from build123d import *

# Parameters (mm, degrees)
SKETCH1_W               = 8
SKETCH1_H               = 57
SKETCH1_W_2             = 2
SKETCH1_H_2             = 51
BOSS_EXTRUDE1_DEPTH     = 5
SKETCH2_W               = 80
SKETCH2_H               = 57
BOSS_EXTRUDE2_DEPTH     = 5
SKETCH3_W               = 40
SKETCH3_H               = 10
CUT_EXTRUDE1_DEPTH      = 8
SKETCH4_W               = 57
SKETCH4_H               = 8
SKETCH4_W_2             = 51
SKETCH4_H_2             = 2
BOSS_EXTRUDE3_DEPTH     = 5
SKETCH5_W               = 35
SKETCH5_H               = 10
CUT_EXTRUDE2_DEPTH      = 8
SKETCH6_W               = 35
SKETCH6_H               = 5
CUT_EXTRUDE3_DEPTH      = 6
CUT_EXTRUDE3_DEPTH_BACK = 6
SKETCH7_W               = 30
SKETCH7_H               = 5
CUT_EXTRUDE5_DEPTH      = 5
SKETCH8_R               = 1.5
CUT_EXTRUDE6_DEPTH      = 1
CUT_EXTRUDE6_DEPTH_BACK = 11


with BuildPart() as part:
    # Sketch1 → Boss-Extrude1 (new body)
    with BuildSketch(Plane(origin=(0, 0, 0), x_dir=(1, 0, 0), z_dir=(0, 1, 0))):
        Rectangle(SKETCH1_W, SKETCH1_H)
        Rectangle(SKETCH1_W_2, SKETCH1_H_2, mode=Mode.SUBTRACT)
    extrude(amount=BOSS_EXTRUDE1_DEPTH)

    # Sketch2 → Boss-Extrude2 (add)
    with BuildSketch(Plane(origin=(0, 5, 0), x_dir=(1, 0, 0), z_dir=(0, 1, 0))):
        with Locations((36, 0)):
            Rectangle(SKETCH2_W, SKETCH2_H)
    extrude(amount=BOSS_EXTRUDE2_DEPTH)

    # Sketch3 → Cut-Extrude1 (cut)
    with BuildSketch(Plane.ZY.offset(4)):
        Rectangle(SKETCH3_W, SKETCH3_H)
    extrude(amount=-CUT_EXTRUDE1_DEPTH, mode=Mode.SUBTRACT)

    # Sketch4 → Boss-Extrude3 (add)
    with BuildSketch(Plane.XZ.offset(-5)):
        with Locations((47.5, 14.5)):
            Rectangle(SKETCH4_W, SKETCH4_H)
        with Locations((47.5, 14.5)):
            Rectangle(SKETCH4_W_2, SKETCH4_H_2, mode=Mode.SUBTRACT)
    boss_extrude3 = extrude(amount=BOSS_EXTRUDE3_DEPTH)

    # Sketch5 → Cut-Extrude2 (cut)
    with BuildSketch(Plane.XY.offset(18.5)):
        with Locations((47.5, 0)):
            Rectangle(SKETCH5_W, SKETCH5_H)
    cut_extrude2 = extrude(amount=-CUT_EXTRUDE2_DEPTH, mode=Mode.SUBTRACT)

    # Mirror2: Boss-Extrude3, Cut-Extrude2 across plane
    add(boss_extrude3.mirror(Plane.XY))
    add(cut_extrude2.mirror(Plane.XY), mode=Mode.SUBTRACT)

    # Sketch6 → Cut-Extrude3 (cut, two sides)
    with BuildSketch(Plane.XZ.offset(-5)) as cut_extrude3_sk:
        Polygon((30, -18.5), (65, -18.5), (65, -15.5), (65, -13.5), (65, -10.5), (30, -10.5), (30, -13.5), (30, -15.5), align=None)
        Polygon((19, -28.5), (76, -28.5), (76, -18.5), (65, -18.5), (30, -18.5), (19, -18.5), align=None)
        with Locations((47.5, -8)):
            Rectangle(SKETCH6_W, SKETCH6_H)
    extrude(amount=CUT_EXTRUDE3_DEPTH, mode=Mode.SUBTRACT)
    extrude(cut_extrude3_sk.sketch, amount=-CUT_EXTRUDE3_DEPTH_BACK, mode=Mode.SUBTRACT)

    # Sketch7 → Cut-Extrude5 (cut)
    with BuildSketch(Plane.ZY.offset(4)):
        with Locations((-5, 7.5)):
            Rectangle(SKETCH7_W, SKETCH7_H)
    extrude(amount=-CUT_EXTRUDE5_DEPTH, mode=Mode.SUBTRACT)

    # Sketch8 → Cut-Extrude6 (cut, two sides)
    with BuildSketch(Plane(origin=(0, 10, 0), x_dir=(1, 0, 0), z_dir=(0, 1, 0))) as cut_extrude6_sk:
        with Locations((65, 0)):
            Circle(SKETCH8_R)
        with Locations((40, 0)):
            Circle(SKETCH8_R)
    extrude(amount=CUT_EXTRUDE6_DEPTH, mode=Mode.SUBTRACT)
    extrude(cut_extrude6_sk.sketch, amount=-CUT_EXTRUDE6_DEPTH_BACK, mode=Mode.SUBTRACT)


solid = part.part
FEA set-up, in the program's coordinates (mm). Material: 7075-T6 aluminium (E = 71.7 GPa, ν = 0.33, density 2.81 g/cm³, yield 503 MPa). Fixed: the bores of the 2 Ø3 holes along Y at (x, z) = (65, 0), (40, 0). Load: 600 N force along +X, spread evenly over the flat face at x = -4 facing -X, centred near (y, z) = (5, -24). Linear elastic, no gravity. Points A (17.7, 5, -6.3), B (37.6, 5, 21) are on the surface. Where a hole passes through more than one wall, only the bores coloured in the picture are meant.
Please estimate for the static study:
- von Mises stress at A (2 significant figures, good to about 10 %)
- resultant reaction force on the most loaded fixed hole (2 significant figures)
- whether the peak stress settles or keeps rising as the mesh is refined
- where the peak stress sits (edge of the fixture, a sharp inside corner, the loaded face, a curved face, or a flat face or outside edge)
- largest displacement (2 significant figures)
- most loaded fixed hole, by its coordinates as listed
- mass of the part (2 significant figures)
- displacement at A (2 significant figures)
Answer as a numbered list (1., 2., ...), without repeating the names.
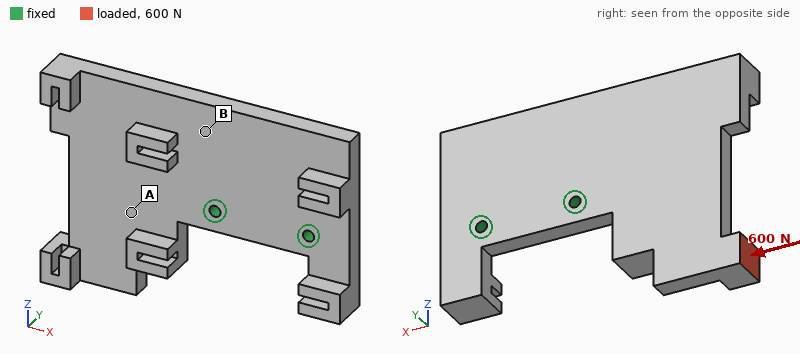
1. 19 MPa
2. 980 N
3. keeps rising
4. edge of the fixture
5. 0.12 mm
6. (40, 0)
7. 53 g
8. 0.028 mm
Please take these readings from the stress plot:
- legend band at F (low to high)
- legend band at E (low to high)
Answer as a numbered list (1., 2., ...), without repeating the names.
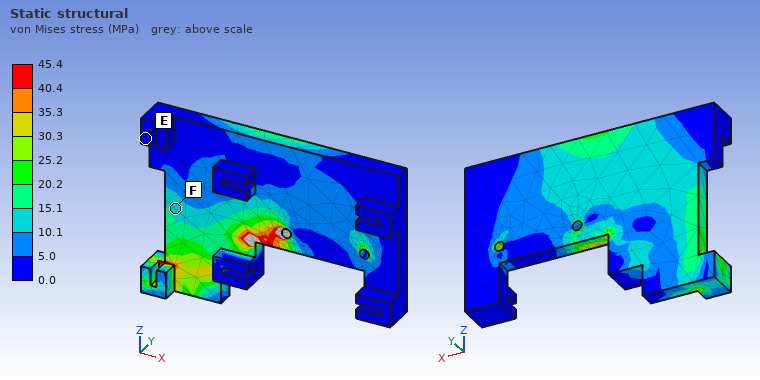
1. 10.1 to 15.1 MPa
2. 0.0 to 5.0 MPa
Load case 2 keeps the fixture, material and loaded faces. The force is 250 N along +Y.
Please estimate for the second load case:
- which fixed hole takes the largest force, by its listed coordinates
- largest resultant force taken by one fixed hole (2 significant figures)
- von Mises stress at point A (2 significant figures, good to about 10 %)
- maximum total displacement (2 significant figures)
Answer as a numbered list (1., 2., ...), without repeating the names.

1. (40, 0)
2. 430 N
3. 53 MPa
4. 0.67 mm
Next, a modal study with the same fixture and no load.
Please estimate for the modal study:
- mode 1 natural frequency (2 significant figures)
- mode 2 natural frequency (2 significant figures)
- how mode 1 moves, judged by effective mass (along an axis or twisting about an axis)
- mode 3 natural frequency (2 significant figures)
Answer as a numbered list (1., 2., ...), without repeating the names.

1. 1500 Hz
2. 1900 Hz
3. along Y
4. 4700 Hz
